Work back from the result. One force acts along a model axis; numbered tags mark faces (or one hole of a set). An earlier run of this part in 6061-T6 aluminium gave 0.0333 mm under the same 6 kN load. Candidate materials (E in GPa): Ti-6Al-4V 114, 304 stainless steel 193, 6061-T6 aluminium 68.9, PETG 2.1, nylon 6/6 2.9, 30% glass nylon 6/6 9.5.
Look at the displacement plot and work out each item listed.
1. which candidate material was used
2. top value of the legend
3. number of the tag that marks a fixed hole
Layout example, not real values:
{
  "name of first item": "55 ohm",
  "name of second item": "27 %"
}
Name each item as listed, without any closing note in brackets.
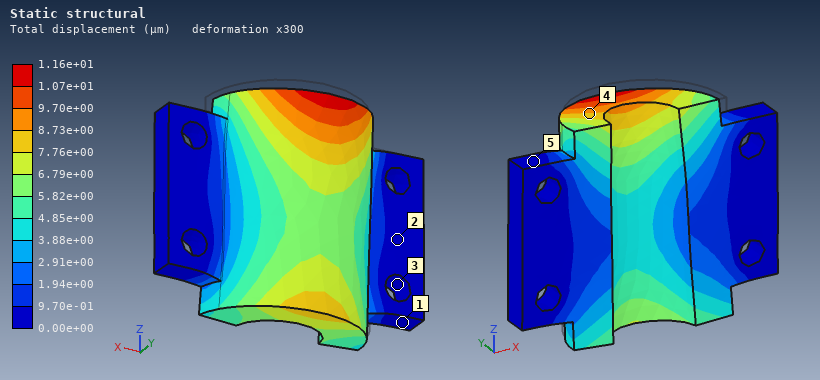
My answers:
{
  "which candidate material was used": "304 stainless steel",
  "top value of the legend": "1.16e+01 µm",
  "number of the tag that marks a fixed hole": "3"
}
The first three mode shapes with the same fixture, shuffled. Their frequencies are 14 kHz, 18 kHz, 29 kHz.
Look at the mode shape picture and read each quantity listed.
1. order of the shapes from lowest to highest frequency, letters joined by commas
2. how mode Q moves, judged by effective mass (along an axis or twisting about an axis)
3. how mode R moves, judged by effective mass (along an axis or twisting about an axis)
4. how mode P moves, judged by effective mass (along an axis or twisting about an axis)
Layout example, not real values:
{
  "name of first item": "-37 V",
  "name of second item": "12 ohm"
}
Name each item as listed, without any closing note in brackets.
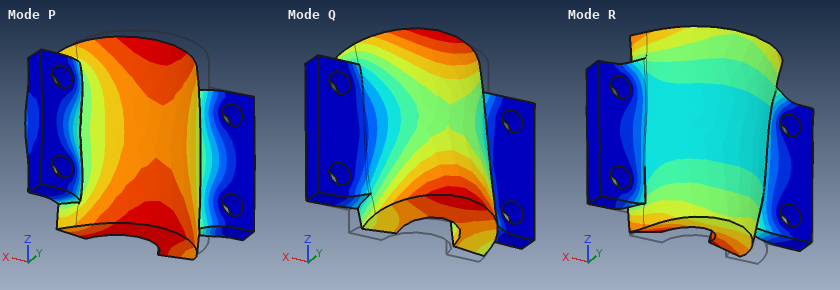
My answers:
{
  "order of the shapes from lowest to highest frequency, letters joined by commas": "Q, P, R",
  "how mode Q moves, judged by effective mass": "along Z",
  "how mode R moves, judged by effective mass": "along Z",
  "how mode P moves, judged by effective mass": "along Y"
}
